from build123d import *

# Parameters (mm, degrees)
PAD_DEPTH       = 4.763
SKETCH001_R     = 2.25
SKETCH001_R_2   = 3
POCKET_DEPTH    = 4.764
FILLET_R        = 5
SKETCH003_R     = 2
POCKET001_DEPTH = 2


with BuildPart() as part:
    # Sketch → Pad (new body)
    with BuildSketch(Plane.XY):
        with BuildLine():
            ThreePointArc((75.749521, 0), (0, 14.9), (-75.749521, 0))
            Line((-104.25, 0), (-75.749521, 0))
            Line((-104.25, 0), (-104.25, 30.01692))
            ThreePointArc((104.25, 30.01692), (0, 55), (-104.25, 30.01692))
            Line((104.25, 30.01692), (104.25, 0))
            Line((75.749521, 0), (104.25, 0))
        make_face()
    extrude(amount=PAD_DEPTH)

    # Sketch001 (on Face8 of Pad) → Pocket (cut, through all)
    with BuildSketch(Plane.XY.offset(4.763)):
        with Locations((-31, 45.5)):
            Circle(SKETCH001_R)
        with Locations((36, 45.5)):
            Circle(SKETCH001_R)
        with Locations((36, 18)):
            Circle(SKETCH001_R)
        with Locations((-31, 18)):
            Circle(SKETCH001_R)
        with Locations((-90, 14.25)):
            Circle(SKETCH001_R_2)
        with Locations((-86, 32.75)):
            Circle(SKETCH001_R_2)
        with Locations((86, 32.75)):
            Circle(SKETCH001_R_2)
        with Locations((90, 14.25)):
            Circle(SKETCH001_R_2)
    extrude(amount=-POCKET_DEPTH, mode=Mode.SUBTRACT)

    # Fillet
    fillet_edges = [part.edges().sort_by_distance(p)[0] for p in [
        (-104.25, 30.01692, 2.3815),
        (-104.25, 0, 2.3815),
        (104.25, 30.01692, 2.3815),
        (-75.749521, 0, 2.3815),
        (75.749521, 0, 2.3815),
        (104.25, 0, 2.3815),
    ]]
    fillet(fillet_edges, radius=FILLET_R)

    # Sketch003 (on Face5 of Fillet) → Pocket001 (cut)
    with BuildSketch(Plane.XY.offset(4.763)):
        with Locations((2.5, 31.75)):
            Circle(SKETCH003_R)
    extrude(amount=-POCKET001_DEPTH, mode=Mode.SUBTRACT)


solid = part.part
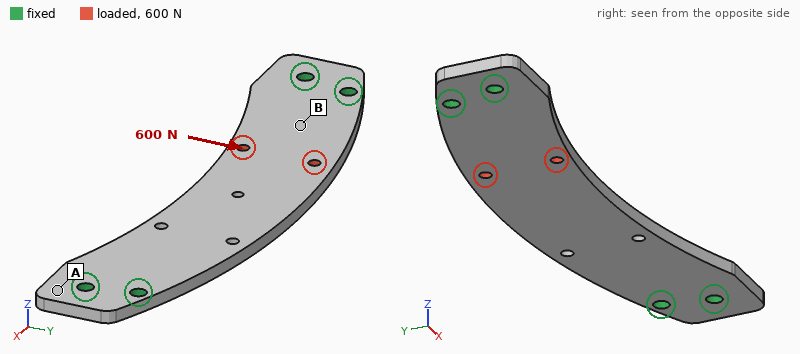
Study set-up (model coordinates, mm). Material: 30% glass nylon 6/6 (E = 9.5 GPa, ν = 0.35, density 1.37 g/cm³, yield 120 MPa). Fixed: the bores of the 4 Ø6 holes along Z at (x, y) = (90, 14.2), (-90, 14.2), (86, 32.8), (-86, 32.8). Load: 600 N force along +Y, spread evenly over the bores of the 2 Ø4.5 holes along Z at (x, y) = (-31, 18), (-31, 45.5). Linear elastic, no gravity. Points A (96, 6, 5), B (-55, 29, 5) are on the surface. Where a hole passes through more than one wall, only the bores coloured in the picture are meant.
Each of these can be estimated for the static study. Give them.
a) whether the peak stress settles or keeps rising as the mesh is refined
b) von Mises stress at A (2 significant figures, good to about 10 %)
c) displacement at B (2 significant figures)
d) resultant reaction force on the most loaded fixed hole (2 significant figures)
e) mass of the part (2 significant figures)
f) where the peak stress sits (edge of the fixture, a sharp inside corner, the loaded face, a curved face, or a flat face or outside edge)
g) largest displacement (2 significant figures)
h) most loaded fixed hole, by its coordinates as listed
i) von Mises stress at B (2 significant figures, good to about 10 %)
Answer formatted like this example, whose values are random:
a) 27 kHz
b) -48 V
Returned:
a) keeps rising
b) 1.9 MPa
c) 53 µm
d) 660 N
e) 53 g
f) edge of the fixture
g) 96 µm
h) (-90, 14.2)
i) 5.5 MPa
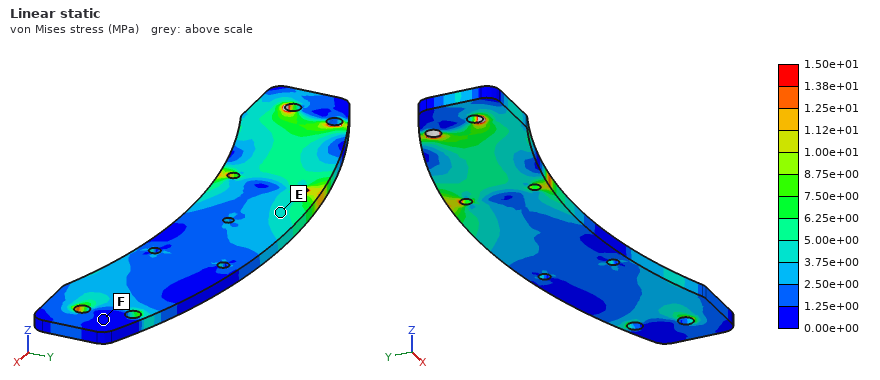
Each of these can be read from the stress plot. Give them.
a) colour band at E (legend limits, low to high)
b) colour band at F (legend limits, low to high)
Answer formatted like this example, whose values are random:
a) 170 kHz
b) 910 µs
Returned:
a) 3.75e+00 to 5.00e+00 MPa
b) 0.00e+00 to 1.25e+00 MPa
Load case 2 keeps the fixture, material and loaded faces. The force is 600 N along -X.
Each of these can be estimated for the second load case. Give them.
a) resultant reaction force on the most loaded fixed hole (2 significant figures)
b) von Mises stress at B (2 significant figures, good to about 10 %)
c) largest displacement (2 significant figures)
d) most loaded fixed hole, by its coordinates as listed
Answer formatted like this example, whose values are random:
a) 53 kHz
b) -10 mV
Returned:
a) 240 N
b) 2.2 MPa
c) 17 µm
d) (-86, 32.8)
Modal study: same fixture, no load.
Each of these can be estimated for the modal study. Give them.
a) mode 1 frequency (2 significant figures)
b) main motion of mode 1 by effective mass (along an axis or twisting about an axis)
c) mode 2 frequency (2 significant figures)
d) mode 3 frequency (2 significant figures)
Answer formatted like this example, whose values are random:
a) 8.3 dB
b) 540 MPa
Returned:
a) 430 Hz
b) along Z
c) 1200 Hz
d) 1200 Hz
